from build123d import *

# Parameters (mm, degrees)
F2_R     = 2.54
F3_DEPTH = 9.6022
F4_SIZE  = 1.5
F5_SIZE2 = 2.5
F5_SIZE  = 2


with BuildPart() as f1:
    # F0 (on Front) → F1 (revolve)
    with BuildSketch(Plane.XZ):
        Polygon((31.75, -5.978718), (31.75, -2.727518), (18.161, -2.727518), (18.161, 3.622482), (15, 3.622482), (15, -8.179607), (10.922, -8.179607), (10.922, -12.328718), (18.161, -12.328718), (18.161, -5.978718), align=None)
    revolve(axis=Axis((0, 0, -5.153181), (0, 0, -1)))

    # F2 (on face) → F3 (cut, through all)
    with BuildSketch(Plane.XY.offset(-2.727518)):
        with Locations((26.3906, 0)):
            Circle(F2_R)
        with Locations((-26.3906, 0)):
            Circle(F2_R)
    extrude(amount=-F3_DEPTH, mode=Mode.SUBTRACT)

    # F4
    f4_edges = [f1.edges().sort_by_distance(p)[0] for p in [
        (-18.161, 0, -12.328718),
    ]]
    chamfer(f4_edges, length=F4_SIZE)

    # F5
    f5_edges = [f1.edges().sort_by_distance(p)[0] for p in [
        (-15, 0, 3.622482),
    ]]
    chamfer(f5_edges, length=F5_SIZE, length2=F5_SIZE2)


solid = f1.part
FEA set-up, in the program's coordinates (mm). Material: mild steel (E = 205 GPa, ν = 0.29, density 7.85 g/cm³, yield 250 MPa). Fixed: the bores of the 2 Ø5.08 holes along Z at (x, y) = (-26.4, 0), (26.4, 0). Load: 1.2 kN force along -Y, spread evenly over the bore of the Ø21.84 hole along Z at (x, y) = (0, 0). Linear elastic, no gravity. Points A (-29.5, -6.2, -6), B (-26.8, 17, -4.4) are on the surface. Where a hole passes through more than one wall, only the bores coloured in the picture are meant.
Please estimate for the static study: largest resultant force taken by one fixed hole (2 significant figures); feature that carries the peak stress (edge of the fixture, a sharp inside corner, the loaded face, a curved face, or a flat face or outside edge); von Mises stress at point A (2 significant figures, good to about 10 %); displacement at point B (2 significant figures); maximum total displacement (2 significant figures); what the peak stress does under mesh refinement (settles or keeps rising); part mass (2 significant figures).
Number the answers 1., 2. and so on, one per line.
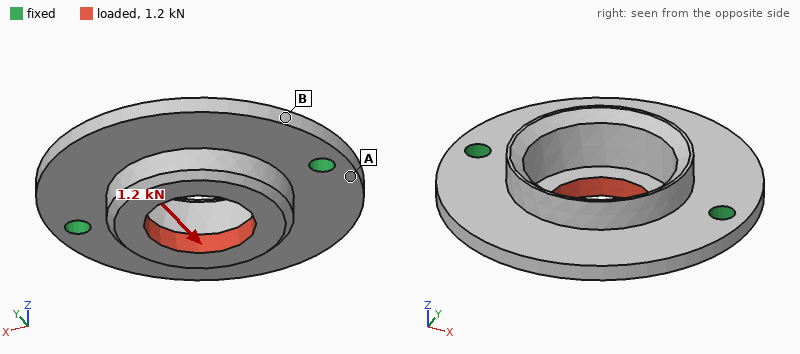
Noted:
1. 600 N
2. edge of the fixture
3. 41 MPa
4. 12 µm
5. 35 µm
6. keeps rising
7. 100 g
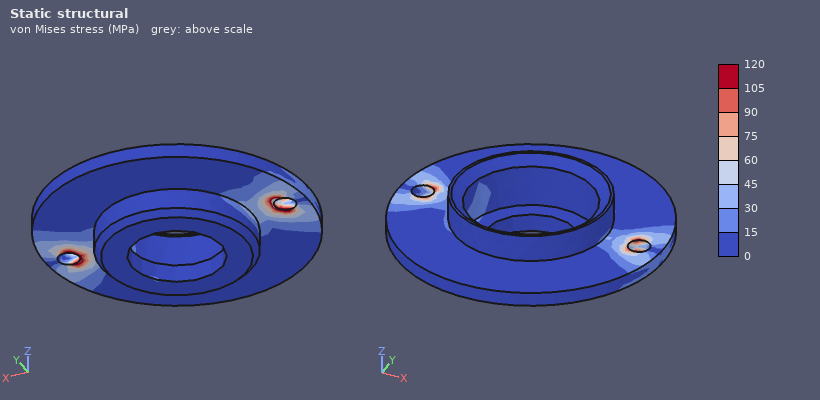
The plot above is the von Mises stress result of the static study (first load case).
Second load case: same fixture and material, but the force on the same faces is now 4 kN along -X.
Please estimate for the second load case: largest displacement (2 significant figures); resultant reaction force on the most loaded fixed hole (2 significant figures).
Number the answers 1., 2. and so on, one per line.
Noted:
1. 6.8 µm
2. 2.1 kN
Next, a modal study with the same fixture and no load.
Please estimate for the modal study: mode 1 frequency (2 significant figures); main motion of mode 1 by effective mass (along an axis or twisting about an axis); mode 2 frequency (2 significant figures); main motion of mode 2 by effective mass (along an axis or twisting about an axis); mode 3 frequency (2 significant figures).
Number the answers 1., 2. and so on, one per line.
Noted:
1. 2600 Hz
2. twisting about X
3. 5000 Hz
4. along Z
5. 9300 Hz
